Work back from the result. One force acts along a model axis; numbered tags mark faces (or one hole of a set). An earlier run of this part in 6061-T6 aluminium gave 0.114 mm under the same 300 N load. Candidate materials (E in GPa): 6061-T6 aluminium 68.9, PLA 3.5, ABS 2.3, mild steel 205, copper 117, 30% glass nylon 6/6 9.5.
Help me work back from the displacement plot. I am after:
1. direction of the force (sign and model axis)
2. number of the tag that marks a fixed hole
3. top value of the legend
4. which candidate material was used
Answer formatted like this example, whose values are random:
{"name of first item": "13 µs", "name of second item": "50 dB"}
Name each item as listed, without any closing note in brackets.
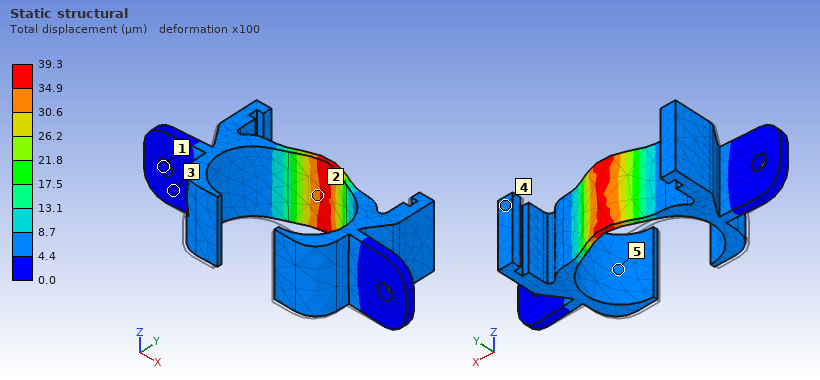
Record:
{"direction of the force": "+Y", "number of the tag that marks a fixed hole": "1", "top value of the legend": "39.3 µm", "which candidate material was used": "mild steel"}
